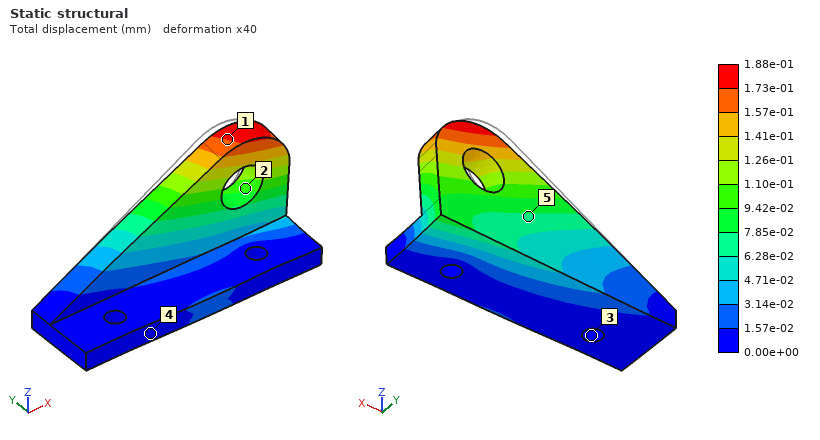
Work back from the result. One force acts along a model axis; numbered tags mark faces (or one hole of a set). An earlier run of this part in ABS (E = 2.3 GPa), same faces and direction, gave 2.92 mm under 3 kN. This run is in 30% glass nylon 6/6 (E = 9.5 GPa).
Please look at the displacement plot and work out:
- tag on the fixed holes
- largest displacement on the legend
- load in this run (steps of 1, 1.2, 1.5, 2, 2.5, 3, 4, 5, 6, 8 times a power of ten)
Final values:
3
1.88e-01 mm
800 N
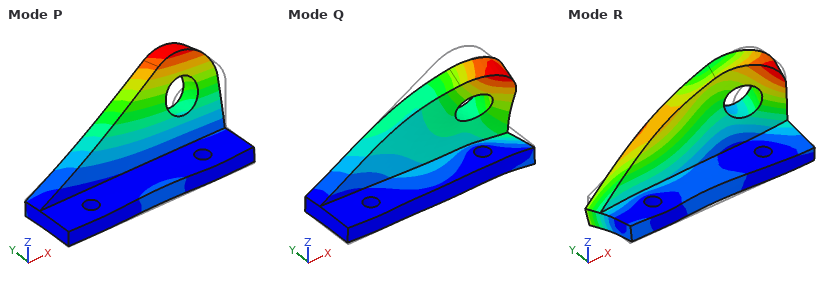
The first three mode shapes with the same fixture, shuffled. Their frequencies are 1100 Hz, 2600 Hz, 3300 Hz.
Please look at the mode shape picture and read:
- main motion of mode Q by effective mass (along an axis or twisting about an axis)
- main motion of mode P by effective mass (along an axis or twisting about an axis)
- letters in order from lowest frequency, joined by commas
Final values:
along Z
along Y
P, R, Q
